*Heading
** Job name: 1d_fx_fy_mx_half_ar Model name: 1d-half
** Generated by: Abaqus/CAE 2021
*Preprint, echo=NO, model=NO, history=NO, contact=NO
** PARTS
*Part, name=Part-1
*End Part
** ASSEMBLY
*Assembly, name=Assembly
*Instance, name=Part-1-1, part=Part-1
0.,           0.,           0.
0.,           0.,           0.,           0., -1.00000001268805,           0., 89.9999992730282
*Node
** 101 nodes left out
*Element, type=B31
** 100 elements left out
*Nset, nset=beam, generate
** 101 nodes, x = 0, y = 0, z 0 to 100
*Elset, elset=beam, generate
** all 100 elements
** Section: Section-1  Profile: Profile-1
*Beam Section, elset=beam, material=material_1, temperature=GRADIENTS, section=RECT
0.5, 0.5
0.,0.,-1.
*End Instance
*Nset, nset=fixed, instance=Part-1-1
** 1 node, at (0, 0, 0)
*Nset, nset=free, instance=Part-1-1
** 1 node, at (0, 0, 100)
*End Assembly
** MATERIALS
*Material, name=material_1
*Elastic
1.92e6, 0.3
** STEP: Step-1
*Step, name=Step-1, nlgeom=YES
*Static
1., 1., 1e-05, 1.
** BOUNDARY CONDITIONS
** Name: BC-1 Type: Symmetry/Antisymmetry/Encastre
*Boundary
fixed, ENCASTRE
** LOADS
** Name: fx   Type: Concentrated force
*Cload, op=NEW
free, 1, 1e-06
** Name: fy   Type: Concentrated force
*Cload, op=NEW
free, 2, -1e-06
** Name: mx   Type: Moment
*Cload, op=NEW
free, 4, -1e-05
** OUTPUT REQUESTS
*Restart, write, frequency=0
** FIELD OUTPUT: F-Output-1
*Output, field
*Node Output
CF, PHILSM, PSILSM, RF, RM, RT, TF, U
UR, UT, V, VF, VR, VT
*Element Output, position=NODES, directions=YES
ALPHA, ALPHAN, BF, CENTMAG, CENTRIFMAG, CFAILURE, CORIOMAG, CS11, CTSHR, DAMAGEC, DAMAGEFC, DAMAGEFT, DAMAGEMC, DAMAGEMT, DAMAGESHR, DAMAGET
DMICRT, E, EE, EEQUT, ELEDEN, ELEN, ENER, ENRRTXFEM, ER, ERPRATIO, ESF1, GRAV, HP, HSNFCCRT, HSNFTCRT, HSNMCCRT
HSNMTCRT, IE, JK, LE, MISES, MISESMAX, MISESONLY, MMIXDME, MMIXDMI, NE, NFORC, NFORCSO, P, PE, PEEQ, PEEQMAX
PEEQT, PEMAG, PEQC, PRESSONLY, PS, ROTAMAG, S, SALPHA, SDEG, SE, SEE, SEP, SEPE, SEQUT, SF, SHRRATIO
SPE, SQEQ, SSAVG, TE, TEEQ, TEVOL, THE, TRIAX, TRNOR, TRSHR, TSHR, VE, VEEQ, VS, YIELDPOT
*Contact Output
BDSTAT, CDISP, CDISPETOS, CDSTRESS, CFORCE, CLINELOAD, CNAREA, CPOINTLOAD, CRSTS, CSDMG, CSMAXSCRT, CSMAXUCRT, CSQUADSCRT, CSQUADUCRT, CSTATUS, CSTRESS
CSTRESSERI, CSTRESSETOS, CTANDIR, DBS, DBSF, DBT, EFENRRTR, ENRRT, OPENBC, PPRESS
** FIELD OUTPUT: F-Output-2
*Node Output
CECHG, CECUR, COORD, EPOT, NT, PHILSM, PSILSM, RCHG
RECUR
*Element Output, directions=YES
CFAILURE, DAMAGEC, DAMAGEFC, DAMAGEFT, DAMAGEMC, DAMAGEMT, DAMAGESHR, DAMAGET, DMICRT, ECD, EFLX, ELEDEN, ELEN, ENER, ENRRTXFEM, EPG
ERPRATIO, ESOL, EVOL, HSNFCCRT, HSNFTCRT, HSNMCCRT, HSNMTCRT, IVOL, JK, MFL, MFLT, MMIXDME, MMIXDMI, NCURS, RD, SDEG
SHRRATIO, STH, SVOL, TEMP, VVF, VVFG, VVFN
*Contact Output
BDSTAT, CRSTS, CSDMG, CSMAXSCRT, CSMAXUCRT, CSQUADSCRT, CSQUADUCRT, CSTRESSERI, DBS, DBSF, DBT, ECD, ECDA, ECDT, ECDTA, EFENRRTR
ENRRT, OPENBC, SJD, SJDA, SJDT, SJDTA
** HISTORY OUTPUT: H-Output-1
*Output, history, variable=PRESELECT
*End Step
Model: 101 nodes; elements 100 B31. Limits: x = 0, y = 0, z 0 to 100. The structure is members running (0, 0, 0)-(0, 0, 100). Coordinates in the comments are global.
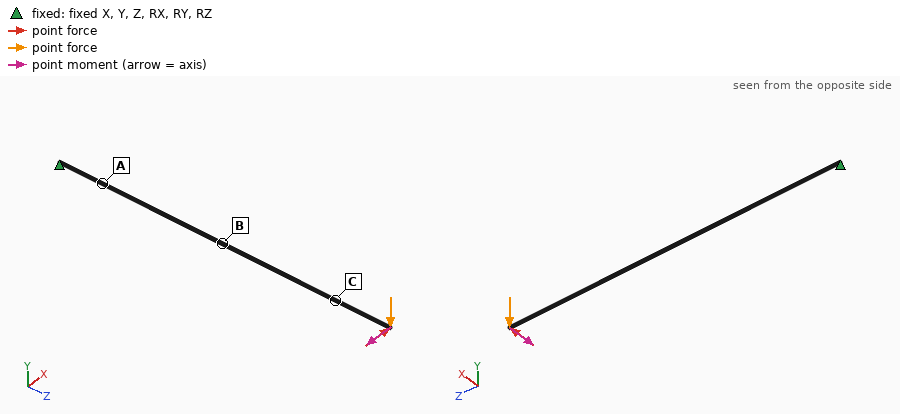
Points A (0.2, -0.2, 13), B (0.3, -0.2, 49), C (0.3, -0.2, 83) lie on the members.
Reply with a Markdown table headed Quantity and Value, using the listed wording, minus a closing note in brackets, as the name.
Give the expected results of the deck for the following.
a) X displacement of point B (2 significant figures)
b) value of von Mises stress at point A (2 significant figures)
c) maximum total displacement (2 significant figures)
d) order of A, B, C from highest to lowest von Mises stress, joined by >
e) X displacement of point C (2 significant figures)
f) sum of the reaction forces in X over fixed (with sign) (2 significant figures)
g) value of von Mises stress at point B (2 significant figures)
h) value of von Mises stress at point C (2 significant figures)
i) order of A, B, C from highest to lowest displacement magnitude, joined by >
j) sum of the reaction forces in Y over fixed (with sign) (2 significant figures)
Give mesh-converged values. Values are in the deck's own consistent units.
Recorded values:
| Quantity | Value |
|---|---|
| X displacement of point B | 1.0e-05 |
| value of von Mises stress at point A | 0.0079 |
| maximum total displacement | 4.4e-05 |
| order of A, B, C from highest to lowest von Mises stress, joined by > | A > B > C |
| X displacement of point C | 2.5e-05 |
| sum of the reaction forces in X over fixed (with sign) | -1.0e-06 |
| value of von Mises stress at point B | 0.0044 |
| value of von Mises stress at point C | 0.0012 |
| order of A, B, C from highest to lowest displacement magnitude, joined by > | C > B > A |
| sum of the reaction forces in Y over fixed (with sign) | 1.0e-06 |
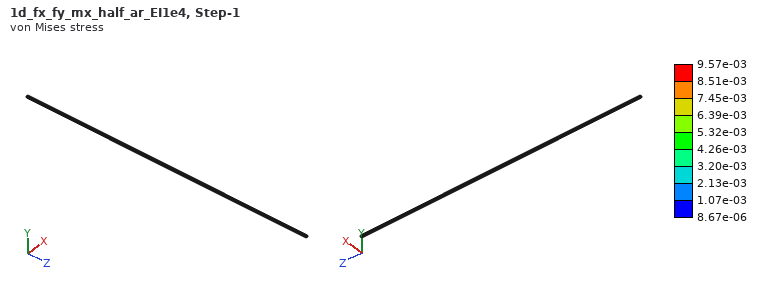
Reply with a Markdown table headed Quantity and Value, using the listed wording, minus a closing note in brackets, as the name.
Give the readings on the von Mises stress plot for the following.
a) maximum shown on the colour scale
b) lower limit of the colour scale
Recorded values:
| Quantity | Value |
|---|---|
| maximum shown on the colour scale | 9.57e-03 |
| lower limit of the colour scale | 8.67e-06 |
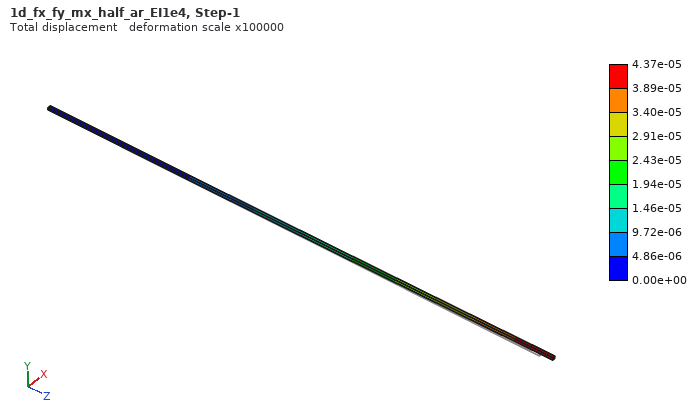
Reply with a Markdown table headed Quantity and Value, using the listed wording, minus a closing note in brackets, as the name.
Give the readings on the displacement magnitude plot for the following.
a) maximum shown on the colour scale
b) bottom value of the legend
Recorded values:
| Quantity | Value |
|---|---|
| maximum shown on the colour scale | 4.37e-05 |
| bottom value of the legend | 0.00e+00 |
